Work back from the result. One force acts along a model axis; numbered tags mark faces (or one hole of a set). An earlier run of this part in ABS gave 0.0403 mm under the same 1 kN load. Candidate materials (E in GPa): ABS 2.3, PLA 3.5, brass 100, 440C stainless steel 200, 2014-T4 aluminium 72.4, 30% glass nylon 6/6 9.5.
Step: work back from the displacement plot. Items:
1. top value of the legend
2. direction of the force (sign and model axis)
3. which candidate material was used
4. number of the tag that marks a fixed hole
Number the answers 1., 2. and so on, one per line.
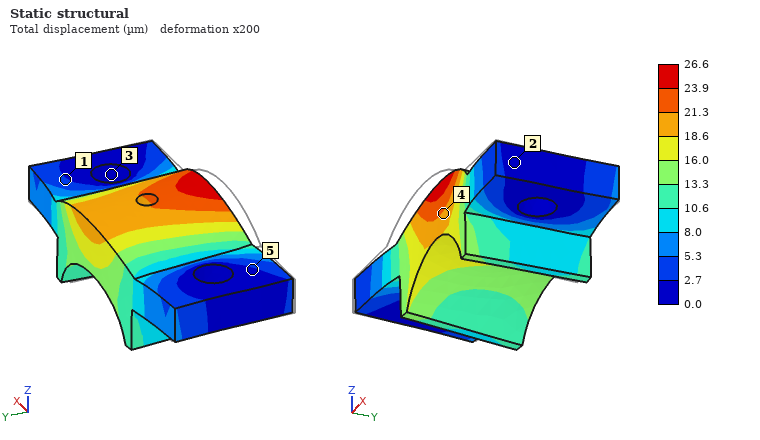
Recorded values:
1. 26.6 µm
2. +Y
3. PLA
4. 3
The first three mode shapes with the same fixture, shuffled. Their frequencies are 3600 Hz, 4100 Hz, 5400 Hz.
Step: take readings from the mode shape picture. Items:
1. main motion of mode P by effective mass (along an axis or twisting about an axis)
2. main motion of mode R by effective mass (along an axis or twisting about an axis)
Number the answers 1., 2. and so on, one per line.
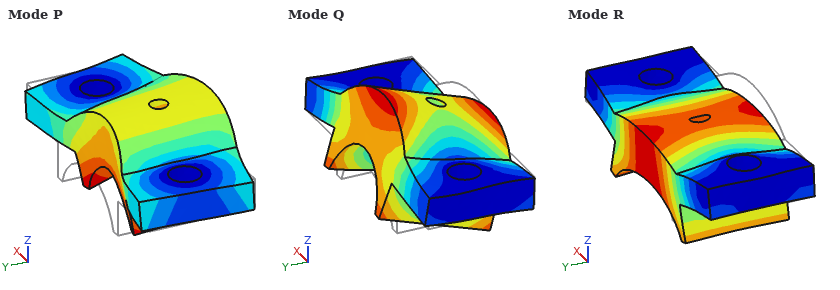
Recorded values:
1. along Y
2. along Z
